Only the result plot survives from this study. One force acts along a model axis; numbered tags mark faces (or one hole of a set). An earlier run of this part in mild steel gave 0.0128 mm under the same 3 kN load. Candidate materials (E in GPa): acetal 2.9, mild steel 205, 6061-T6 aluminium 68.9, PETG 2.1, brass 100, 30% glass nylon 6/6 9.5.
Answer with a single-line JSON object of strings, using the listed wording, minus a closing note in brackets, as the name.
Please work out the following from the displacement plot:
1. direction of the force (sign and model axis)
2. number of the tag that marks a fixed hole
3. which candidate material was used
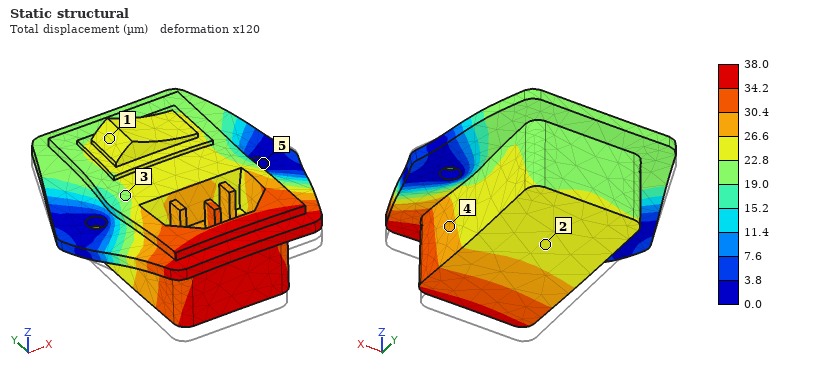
{"direction of the force": "+Z", "number of the tag that marks a fixed hole": "5", "which candidate material was used": "6061-T6 aluminium"}
